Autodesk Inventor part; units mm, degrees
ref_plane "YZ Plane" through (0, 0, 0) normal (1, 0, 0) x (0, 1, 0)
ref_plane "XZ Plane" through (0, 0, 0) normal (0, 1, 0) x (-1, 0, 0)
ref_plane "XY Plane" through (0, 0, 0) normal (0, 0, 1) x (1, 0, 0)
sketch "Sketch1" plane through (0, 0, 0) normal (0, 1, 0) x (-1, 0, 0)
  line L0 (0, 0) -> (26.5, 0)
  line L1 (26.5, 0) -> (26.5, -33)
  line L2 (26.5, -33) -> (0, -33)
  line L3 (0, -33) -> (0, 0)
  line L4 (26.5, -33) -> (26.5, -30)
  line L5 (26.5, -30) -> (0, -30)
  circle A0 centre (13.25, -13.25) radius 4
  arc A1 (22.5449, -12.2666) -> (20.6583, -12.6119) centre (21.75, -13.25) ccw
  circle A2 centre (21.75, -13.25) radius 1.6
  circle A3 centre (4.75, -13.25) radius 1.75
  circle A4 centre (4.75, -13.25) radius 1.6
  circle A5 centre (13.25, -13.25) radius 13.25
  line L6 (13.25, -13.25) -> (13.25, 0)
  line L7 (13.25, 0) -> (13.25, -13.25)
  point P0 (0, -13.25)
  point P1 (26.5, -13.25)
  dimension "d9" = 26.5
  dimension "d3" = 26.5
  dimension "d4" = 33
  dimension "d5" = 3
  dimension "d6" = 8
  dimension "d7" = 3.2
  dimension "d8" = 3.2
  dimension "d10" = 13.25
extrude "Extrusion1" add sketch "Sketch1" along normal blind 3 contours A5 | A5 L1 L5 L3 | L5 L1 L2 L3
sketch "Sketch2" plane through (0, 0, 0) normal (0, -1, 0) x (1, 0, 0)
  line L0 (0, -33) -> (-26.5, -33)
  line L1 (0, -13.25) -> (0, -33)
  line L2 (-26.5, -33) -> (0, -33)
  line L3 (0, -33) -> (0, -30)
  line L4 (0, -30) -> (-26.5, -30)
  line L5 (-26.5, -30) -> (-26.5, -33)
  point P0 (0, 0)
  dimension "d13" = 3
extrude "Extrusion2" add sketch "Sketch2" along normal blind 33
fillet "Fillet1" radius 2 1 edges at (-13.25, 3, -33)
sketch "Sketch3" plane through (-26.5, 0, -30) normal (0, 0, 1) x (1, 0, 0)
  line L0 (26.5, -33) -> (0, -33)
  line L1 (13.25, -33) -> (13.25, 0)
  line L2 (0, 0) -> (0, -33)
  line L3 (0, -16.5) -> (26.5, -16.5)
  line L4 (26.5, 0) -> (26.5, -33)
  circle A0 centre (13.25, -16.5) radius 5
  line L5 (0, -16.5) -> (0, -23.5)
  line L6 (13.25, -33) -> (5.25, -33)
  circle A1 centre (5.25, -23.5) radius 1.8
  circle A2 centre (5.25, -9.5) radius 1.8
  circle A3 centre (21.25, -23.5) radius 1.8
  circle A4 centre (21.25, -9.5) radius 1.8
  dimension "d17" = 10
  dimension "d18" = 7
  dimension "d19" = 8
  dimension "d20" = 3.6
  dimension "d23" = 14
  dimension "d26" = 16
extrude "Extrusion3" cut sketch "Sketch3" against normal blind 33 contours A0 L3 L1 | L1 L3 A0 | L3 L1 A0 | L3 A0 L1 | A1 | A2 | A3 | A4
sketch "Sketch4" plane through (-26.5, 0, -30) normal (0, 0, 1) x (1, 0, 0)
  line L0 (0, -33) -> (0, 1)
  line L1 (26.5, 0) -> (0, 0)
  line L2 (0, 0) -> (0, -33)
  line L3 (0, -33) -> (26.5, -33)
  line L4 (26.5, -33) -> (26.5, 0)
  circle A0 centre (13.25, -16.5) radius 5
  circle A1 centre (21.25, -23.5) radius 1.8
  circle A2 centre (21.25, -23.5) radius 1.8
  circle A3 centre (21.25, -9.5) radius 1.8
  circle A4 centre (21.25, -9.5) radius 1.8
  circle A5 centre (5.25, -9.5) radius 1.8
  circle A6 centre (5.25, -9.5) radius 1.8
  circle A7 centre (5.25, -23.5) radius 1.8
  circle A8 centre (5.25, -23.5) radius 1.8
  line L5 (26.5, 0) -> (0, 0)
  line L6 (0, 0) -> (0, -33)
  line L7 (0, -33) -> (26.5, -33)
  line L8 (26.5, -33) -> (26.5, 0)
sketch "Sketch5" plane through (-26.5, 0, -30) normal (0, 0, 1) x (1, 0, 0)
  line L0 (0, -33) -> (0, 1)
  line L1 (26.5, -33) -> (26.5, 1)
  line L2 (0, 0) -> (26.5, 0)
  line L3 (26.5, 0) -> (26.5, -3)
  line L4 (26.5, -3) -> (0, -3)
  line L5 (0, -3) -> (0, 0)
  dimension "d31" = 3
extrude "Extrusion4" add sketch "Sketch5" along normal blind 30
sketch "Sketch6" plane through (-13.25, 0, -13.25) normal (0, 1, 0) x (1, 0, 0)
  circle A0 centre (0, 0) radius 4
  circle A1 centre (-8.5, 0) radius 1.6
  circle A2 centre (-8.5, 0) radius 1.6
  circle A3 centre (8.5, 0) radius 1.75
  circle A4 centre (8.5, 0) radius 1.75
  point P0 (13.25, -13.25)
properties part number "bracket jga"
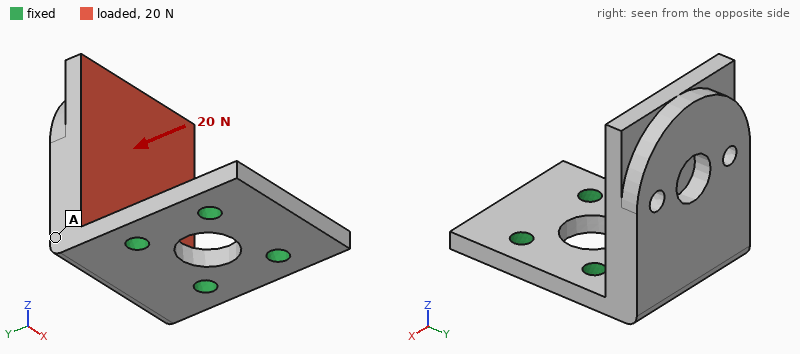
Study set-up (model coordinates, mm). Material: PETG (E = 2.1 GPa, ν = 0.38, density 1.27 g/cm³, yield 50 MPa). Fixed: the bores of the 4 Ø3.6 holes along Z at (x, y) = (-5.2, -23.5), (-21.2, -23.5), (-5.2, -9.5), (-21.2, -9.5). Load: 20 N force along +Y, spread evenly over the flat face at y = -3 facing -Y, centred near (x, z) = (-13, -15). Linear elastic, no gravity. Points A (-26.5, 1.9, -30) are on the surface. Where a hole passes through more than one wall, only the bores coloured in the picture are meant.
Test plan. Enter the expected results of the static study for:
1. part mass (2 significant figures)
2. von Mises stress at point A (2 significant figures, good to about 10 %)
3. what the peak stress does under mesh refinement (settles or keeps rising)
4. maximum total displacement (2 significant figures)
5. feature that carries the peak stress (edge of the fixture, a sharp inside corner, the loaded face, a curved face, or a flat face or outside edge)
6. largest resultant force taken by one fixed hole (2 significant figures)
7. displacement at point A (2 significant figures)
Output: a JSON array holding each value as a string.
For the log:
["8.7 g", "1.3 MPa", "keeps rising", "0.65 mm", "edge of the fixture", "10 N", "0.13 mm"]
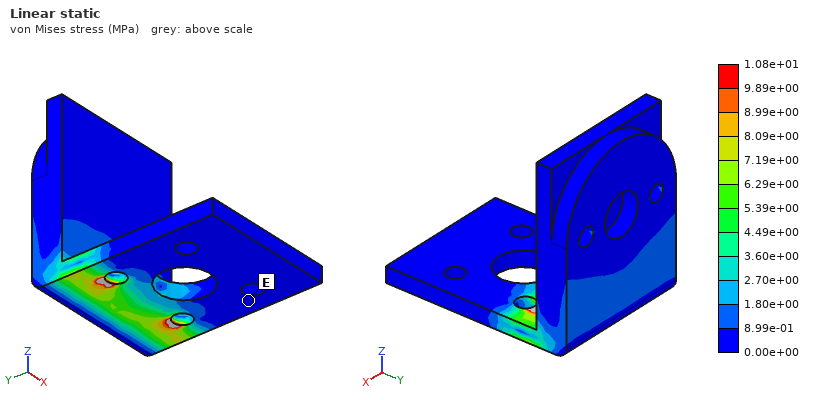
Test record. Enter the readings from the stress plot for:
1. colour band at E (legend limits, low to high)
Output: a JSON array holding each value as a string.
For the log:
["0.00e+00 to 8.99e-01 MPa"]
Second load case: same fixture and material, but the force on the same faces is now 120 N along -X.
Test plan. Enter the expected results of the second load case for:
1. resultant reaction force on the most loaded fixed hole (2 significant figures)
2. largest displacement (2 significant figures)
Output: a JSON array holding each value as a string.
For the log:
["130 N", "0.61 mm"]
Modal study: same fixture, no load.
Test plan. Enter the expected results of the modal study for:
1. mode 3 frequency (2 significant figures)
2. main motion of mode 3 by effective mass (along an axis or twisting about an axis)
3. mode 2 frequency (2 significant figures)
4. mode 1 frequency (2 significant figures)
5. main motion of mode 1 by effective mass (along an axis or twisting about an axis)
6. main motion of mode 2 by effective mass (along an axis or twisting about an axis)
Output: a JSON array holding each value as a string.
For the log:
["2700 Hz", "along Z", "1200 Hz", "470 Hz", "along Y", "along X"]
